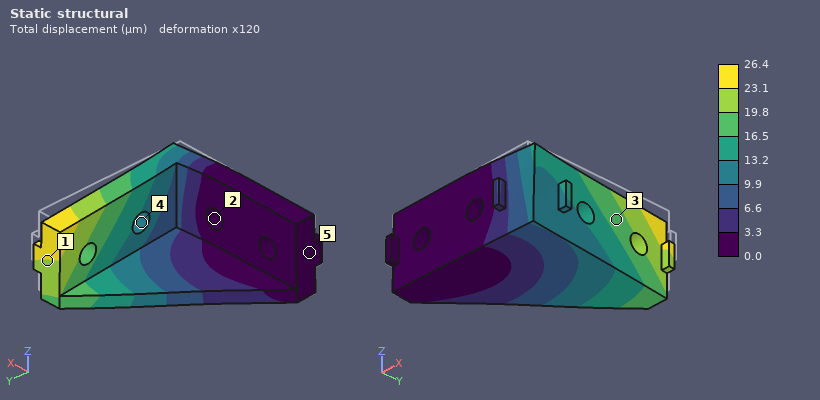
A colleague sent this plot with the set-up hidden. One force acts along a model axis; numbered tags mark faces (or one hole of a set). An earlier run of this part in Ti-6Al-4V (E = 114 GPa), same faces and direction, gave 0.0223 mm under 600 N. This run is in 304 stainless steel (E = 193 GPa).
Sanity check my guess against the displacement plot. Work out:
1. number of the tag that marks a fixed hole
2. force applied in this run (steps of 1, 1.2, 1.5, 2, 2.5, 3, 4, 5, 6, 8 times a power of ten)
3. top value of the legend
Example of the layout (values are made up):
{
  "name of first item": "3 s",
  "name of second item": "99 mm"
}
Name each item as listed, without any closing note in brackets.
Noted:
{
  "number of the tag that marks a fixed hole": "2",
  "force applied in this run": "1.2 kN",
  "top value of the legend": "26.4 µm"
}
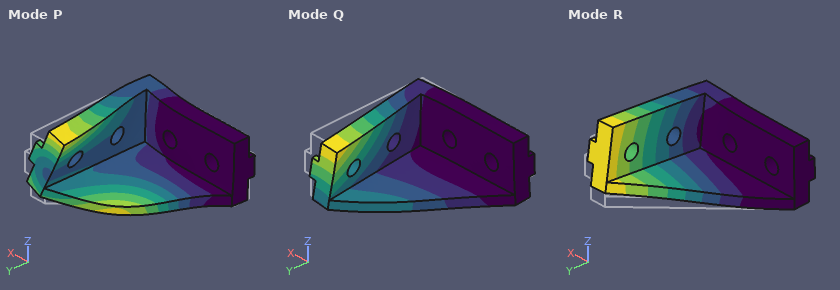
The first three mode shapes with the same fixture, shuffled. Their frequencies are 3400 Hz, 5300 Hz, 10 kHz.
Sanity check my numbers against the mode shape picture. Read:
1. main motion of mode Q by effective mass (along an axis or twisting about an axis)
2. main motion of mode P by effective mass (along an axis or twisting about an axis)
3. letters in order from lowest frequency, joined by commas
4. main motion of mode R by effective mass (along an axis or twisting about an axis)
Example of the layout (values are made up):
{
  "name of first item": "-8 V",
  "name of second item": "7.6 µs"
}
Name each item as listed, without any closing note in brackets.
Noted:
{
  "main motion of mode Q by effective mass": "along X",
  "main motion of mode P by effective mass": "along Y",
  "letters in order from lowest frequency, joined by commas": "R, Q, P",
  "main motion of mode R by effective mass": "along Z"
}
